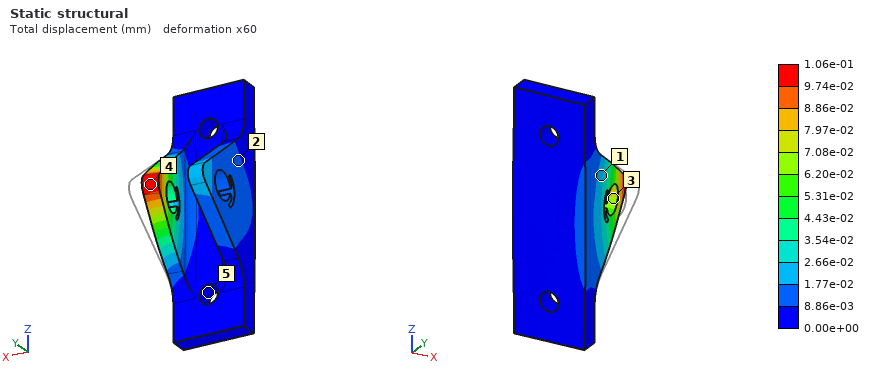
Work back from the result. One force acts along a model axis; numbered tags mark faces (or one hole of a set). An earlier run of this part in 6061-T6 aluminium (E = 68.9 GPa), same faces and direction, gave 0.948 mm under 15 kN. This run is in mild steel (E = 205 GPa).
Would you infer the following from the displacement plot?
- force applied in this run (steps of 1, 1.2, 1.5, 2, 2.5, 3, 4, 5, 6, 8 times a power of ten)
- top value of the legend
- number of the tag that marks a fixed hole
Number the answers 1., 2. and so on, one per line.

1. 5 kN
2. 1.06e-01 mm
3. 5
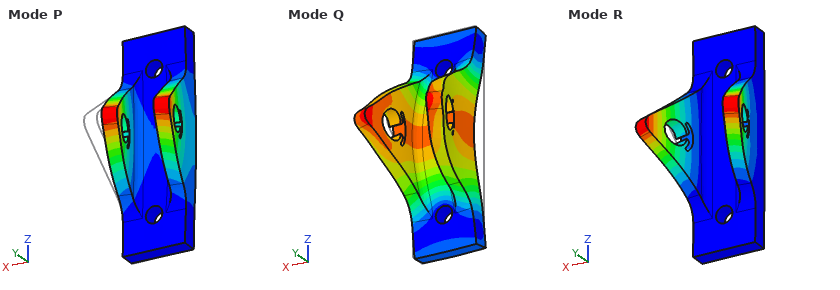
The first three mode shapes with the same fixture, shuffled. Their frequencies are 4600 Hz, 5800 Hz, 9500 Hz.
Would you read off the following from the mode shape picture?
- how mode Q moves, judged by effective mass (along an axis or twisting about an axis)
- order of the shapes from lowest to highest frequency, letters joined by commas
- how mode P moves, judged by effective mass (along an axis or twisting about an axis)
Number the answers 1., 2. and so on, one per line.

1. along Y
2. P, R, Q
3. along X
